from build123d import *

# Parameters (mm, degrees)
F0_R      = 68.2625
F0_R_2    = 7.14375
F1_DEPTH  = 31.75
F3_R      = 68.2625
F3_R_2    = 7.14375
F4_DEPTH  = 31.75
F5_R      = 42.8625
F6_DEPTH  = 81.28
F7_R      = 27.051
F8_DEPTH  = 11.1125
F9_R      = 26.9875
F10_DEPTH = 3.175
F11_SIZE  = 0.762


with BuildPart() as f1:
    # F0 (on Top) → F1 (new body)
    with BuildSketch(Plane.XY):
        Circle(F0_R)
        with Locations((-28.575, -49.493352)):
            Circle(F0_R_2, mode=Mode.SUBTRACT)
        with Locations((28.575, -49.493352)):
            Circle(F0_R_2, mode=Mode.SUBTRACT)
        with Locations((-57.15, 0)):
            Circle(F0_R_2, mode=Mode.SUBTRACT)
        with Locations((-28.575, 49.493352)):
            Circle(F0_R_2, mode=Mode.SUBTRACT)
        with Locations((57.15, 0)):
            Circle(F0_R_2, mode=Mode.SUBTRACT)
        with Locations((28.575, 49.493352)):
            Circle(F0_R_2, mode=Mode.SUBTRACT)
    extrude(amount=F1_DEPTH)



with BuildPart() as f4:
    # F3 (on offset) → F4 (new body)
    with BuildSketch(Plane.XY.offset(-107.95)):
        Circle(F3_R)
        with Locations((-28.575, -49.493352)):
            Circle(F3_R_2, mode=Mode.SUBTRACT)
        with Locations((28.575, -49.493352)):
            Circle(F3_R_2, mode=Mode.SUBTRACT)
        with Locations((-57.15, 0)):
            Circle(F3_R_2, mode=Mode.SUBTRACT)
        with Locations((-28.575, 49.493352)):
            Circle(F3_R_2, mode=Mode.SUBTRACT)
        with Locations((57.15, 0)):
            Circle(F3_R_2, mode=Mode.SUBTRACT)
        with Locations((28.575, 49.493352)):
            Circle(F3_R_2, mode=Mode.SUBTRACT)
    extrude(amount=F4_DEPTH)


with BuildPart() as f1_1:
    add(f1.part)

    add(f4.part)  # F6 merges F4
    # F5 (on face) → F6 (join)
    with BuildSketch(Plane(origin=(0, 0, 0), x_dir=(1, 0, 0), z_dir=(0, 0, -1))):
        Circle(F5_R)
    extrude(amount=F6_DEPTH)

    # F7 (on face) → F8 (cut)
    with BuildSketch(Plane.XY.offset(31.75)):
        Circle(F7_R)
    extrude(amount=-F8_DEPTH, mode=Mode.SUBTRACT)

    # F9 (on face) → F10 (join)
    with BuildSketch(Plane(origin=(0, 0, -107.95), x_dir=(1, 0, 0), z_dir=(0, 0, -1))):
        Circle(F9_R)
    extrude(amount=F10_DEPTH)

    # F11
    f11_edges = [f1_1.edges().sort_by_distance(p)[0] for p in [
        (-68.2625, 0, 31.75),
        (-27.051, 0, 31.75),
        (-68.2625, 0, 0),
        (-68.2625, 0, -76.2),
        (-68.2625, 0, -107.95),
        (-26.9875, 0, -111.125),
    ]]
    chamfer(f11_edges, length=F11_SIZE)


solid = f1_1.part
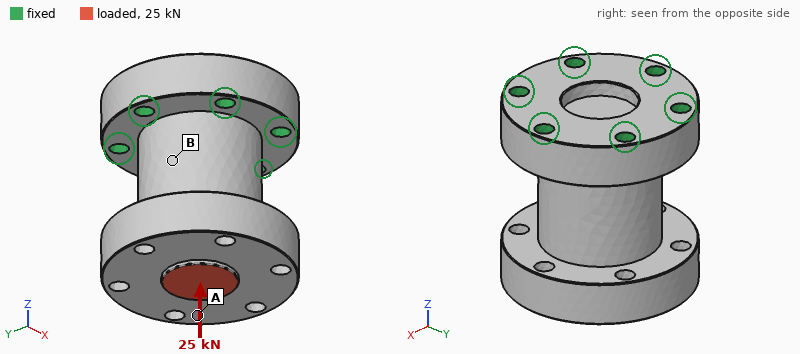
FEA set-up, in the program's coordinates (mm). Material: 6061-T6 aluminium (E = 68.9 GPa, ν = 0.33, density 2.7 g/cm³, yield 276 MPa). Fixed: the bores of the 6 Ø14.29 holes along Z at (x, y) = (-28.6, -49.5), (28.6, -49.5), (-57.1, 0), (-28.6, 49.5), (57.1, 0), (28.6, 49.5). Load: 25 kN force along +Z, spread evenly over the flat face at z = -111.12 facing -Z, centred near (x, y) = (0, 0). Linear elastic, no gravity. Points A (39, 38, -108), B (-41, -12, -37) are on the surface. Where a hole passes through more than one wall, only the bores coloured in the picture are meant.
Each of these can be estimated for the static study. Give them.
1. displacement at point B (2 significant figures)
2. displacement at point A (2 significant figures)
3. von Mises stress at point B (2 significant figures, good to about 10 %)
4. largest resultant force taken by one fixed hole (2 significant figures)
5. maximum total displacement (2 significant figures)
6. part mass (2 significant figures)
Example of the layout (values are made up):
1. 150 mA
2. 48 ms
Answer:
1. 5.9 µm
2. 8.1 µm
3. 4.4 MPa
4. 4.6 kN
5. 13 µm
6. 3.5 kg
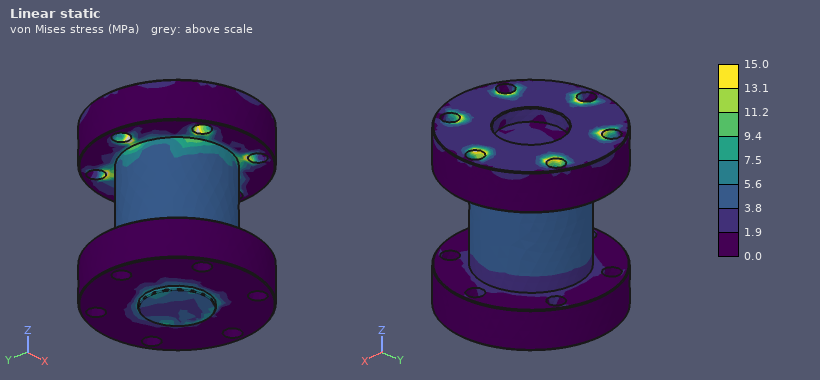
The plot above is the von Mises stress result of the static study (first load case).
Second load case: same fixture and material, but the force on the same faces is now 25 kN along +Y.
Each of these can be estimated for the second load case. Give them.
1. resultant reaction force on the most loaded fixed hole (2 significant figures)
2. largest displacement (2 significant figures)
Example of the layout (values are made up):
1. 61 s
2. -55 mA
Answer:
1. 19 kN
2. 0.14 mm
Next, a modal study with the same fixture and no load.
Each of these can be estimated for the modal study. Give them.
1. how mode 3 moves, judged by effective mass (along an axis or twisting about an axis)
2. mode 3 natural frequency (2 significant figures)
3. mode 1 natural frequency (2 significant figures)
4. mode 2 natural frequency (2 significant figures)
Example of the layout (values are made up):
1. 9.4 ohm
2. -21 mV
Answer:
1. twisting about Z
2. 3400 Hz
3. 2200 Hz
4. 2200 Hz
